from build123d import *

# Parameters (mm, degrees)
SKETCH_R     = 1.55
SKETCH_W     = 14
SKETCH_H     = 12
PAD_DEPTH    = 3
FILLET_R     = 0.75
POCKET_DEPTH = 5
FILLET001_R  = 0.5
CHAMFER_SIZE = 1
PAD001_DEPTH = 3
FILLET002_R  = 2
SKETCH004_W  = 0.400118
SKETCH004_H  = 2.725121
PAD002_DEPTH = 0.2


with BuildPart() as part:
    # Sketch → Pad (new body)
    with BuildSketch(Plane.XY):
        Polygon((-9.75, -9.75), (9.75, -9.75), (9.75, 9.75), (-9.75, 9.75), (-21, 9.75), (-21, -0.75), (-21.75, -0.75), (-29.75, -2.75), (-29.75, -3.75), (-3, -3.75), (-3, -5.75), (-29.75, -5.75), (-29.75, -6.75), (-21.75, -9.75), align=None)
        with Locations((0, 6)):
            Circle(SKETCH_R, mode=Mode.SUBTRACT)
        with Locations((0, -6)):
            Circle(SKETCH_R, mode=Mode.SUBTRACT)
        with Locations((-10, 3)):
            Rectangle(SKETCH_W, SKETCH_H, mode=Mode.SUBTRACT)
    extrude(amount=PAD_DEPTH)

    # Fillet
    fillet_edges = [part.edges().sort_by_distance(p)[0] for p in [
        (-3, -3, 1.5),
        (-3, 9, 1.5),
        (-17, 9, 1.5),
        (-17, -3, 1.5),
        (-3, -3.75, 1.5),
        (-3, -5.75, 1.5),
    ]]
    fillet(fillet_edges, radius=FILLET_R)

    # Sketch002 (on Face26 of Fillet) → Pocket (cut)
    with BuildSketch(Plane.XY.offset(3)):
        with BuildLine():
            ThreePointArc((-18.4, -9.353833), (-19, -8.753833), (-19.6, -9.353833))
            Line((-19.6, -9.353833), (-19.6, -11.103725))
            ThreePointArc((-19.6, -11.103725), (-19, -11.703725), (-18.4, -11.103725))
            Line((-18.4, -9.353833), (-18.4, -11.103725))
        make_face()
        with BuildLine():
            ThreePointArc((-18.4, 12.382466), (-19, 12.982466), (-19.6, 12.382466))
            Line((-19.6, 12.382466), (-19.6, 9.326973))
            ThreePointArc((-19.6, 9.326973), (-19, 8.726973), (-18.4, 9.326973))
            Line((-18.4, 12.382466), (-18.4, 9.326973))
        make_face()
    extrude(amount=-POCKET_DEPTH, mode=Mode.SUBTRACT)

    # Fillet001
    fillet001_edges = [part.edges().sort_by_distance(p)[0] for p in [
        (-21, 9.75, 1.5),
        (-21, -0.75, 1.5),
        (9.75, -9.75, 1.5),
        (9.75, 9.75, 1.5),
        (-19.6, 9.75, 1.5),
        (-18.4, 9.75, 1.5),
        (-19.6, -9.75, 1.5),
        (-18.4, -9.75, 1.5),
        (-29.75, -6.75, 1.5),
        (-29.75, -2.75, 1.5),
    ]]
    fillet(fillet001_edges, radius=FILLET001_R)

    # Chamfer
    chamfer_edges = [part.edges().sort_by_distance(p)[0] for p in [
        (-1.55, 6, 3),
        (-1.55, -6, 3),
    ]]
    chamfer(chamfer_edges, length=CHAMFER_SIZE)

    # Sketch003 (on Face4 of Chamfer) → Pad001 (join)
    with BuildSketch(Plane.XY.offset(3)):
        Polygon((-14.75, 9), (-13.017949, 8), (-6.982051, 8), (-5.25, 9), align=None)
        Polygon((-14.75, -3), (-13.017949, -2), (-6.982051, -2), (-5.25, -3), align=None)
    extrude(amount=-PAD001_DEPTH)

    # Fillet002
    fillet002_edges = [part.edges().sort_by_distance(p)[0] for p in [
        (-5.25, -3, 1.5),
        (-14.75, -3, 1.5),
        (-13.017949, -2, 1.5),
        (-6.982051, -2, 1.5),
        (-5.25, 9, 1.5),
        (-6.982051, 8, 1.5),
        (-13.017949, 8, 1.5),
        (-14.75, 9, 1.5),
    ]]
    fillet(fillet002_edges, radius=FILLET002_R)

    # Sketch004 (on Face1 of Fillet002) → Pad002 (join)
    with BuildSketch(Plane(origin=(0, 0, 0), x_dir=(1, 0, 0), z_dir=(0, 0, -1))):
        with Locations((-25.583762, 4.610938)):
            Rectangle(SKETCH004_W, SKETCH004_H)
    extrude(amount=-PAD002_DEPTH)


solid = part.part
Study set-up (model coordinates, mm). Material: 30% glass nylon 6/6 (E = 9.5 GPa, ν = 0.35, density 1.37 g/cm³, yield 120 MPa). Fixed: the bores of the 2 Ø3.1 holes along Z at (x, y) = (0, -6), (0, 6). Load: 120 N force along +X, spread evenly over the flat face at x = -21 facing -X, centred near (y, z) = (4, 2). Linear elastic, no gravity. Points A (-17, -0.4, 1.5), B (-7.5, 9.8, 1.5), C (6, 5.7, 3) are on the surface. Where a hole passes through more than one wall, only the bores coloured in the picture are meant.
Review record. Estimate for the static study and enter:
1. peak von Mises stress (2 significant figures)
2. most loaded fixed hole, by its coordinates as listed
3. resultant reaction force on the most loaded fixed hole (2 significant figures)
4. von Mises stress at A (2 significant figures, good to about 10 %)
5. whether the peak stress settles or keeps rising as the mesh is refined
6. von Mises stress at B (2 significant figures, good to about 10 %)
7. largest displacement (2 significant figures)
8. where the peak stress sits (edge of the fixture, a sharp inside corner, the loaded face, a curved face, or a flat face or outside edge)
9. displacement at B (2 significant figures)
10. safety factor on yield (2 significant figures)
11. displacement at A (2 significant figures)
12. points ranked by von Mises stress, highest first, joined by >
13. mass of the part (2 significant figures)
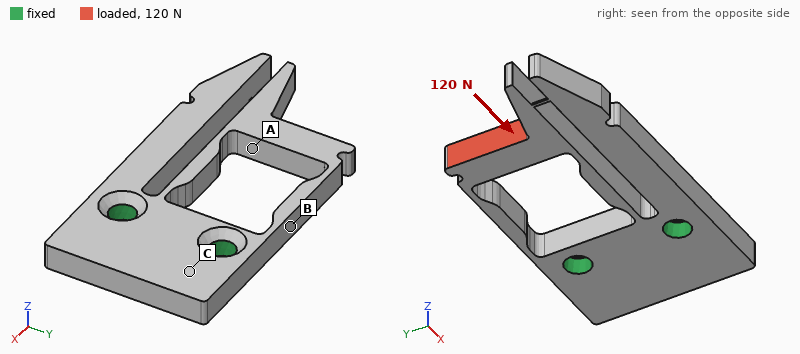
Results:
75 MPa
(0, 6)
90 N
16 MPa
settles
32 MPa
79 µm
a curved face
26 µm
1.6
65 µm
B > A > C
1.8 g
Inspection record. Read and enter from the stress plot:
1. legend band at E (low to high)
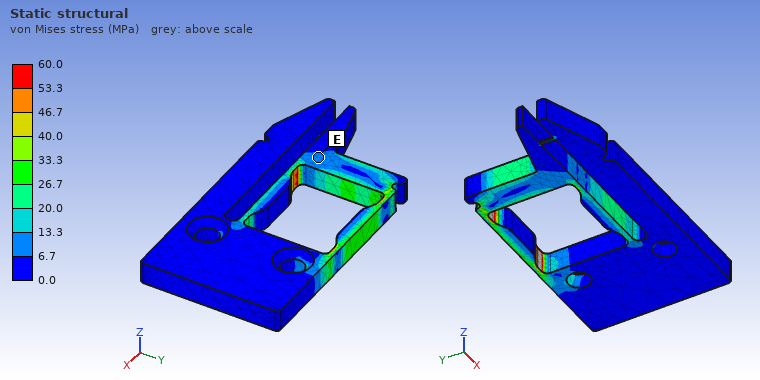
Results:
6.7 to 13.3 MPa
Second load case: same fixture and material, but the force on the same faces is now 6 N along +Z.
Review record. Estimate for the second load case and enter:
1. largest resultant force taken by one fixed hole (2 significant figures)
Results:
3.2 N
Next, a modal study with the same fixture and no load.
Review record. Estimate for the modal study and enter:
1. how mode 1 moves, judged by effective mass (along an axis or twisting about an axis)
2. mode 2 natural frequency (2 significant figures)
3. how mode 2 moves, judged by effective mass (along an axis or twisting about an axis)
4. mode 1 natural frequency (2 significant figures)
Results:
along Z
1500 Hz
along Y
1300 Hz
